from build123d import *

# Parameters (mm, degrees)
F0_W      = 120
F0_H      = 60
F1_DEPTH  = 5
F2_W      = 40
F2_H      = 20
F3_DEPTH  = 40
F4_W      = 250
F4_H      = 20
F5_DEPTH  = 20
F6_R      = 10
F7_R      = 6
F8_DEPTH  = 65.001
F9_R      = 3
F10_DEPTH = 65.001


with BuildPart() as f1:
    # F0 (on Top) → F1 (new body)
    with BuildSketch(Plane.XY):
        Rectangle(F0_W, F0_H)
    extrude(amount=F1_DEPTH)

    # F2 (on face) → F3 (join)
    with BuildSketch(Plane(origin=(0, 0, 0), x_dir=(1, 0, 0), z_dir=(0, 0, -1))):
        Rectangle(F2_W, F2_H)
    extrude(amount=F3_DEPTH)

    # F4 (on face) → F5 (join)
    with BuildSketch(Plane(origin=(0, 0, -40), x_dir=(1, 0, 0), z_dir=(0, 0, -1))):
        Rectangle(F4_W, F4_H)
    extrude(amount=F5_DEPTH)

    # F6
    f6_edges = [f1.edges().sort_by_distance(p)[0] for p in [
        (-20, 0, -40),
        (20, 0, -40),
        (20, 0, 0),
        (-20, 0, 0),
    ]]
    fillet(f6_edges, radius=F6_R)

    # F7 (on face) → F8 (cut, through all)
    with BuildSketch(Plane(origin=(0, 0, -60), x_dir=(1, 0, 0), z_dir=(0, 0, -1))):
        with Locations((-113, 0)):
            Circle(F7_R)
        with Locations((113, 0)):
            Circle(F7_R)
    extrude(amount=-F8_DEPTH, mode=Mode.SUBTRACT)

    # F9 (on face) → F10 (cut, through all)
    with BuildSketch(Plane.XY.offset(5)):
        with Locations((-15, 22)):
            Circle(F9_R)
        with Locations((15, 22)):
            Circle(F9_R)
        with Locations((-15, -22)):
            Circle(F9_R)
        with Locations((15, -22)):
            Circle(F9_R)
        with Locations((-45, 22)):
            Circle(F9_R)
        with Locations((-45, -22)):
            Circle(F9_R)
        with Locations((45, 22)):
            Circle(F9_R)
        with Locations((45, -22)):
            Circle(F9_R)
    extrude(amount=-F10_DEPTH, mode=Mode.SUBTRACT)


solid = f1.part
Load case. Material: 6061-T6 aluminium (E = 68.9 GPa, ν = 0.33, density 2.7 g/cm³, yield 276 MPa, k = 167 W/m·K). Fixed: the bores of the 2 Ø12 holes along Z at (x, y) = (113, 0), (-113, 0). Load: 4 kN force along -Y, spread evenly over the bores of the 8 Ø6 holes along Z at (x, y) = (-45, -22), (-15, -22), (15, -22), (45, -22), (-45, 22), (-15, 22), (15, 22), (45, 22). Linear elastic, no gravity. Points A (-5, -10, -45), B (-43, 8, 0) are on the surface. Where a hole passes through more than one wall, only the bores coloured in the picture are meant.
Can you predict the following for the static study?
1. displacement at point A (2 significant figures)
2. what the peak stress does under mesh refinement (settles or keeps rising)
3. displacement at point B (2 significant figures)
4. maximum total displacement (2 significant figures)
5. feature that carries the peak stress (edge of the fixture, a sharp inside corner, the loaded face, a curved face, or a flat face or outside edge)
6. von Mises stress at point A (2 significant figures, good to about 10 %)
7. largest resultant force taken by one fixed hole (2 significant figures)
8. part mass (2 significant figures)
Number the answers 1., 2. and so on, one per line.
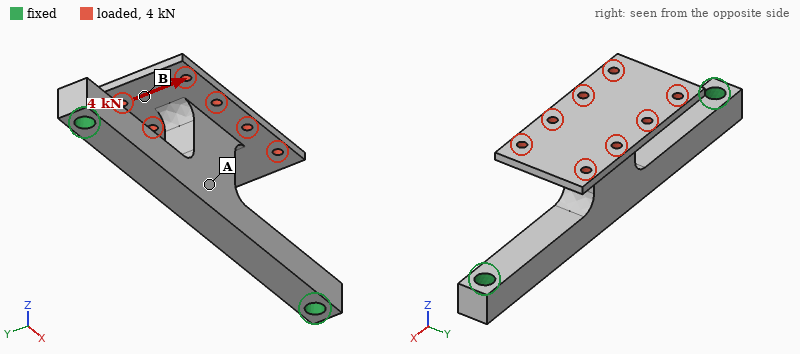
1. 0.36 mm
2. keeps rising
3. 1.1 mm
4. 1.4 mm
5. edge of the fixture
6. 64 MPa
7. 2.0 kN
8. 440 g
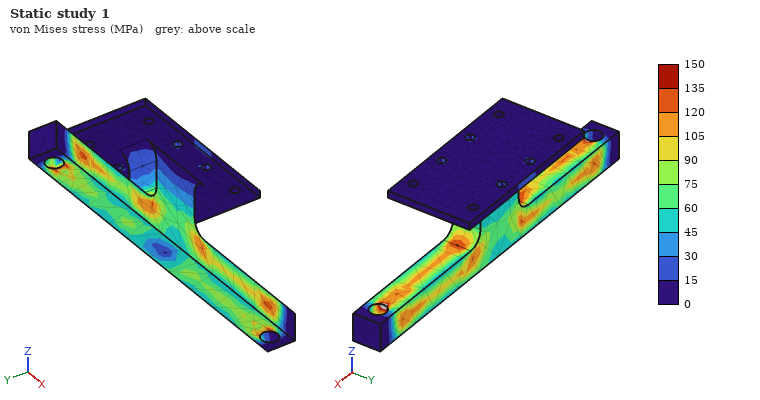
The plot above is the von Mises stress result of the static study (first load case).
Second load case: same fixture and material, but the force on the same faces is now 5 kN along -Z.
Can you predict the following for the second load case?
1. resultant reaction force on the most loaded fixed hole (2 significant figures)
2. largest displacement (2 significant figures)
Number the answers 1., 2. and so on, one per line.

1. 2.7 kN
2. 0.54 mm
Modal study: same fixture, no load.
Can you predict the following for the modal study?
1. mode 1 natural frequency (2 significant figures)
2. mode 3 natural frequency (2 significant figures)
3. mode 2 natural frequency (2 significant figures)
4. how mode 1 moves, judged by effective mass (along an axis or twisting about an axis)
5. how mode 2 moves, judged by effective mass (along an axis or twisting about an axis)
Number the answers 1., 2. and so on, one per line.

1. 760 Hz
2. 1900 Hz
3. 1400 Hz
4. along Y
5. along Z
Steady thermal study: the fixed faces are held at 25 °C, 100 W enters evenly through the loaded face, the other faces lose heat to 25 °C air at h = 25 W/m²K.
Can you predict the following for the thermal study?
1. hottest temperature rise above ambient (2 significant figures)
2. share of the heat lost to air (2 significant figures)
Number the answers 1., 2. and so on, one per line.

1. 82 K
2. 43 %
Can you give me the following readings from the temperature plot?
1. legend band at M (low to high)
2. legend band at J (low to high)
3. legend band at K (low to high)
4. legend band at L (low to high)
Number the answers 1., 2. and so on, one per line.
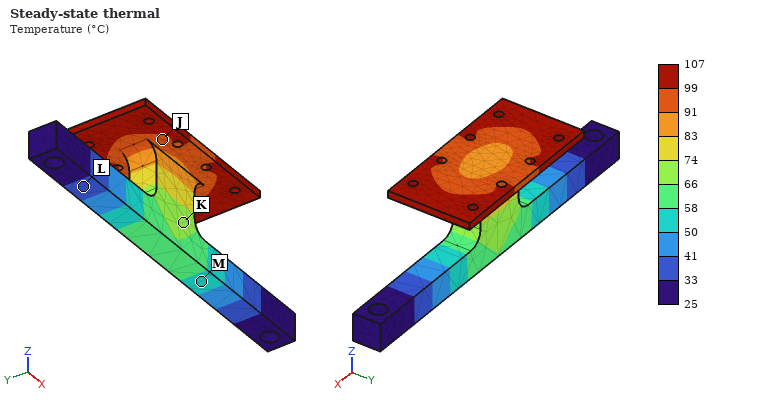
1. 50 to 58 °C
2. 91 to 99 °C
3. 66 to 74 °C
4. 33 to 41 °C
